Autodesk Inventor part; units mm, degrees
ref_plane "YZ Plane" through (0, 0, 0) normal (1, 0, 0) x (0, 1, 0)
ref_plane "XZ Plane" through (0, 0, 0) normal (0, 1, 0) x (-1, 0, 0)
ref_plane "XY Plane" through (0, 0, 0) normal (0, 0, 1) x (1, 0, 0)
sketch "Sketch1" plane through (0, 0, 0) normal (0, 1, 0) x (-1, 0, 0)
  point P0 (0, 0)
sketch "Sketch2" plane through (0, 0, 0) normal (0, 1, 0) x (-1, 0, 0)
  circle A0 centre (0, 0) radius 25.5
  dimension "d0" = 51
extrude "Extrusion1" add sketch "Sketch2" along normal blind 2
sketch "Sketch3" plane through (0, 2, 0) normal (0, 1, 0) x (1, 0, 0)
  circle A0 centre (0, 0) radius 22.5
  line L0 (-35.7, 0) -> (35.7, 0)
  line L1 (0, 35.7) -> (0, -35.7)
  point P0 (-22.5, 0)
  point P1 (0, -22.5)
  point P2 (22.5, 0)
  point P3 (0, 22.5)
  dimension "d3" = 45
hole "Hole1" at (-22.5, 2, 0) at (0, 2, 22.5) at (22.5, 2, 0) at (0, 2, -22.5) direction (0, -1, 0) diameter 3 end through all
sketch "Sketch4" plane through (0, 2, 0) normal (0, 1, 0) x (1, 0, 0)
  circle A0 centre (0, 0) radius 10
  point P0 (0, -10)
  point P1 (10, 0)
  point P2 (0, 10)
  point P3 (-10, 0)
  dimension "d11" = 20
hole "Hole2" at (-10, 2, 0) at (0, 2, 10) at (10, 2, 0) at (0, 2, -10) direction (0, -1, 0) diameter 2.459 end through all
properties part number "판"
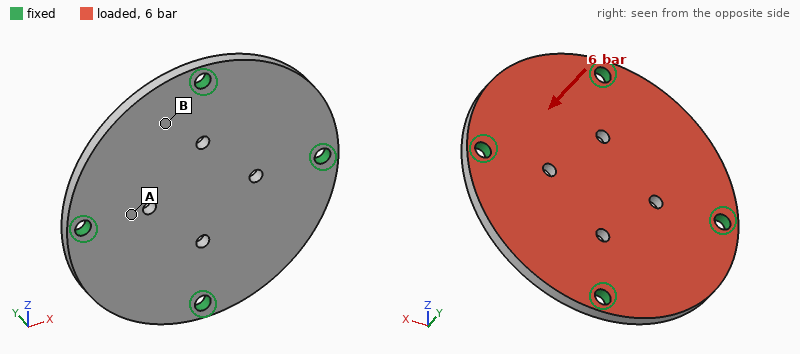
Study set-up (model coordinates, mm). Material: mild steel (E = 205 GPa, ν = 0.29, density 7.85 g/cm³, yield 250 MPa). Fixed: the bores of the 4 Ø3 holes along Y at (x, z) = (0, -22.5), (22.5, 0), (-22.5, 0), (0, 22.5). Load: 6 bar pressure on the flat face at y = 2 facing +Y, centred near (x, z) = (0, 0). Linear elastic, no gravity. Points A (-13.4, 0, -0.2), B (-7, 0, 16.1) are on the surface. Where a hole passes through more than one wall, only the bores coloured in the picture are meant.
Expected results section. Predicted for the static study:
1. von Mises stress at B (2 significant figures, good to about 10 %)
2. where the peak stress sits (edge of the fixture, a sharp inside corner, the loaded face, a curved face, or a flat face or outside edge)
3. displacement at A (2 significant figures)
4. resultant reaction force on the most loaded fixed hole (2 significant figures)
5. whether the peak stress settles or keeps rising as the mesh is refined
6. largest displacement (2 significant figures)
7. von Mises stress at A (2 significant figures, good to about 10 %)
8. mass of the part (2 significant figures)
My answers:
35 MPa
edge of the fixture
13 µm
300 N
keeps rising
25 µm
18 MPa
31 g
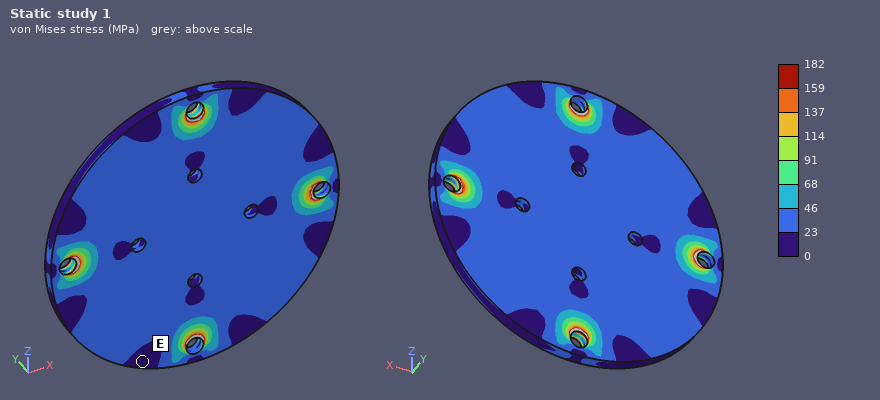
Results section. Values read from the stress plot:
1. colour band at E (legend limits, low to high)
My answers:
0 to 23 MPa
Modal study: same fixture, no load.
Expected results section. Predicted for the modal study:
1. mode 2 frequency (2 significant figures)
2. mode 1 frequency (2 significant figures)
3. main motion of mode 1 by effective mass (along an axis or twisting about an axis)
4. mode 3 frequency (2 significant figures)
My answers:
9100 Hz
7600 Hz
along Y
9400 Hz
